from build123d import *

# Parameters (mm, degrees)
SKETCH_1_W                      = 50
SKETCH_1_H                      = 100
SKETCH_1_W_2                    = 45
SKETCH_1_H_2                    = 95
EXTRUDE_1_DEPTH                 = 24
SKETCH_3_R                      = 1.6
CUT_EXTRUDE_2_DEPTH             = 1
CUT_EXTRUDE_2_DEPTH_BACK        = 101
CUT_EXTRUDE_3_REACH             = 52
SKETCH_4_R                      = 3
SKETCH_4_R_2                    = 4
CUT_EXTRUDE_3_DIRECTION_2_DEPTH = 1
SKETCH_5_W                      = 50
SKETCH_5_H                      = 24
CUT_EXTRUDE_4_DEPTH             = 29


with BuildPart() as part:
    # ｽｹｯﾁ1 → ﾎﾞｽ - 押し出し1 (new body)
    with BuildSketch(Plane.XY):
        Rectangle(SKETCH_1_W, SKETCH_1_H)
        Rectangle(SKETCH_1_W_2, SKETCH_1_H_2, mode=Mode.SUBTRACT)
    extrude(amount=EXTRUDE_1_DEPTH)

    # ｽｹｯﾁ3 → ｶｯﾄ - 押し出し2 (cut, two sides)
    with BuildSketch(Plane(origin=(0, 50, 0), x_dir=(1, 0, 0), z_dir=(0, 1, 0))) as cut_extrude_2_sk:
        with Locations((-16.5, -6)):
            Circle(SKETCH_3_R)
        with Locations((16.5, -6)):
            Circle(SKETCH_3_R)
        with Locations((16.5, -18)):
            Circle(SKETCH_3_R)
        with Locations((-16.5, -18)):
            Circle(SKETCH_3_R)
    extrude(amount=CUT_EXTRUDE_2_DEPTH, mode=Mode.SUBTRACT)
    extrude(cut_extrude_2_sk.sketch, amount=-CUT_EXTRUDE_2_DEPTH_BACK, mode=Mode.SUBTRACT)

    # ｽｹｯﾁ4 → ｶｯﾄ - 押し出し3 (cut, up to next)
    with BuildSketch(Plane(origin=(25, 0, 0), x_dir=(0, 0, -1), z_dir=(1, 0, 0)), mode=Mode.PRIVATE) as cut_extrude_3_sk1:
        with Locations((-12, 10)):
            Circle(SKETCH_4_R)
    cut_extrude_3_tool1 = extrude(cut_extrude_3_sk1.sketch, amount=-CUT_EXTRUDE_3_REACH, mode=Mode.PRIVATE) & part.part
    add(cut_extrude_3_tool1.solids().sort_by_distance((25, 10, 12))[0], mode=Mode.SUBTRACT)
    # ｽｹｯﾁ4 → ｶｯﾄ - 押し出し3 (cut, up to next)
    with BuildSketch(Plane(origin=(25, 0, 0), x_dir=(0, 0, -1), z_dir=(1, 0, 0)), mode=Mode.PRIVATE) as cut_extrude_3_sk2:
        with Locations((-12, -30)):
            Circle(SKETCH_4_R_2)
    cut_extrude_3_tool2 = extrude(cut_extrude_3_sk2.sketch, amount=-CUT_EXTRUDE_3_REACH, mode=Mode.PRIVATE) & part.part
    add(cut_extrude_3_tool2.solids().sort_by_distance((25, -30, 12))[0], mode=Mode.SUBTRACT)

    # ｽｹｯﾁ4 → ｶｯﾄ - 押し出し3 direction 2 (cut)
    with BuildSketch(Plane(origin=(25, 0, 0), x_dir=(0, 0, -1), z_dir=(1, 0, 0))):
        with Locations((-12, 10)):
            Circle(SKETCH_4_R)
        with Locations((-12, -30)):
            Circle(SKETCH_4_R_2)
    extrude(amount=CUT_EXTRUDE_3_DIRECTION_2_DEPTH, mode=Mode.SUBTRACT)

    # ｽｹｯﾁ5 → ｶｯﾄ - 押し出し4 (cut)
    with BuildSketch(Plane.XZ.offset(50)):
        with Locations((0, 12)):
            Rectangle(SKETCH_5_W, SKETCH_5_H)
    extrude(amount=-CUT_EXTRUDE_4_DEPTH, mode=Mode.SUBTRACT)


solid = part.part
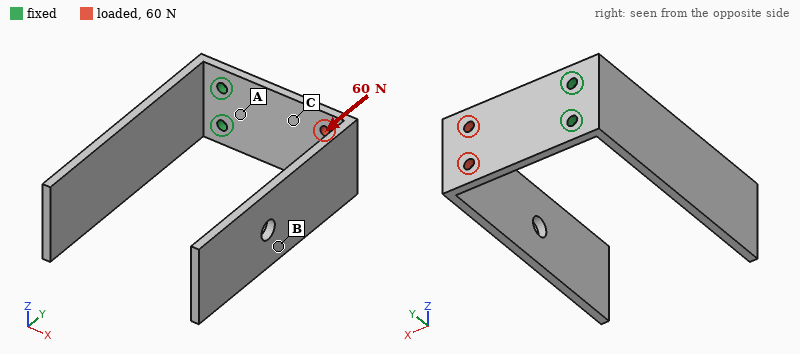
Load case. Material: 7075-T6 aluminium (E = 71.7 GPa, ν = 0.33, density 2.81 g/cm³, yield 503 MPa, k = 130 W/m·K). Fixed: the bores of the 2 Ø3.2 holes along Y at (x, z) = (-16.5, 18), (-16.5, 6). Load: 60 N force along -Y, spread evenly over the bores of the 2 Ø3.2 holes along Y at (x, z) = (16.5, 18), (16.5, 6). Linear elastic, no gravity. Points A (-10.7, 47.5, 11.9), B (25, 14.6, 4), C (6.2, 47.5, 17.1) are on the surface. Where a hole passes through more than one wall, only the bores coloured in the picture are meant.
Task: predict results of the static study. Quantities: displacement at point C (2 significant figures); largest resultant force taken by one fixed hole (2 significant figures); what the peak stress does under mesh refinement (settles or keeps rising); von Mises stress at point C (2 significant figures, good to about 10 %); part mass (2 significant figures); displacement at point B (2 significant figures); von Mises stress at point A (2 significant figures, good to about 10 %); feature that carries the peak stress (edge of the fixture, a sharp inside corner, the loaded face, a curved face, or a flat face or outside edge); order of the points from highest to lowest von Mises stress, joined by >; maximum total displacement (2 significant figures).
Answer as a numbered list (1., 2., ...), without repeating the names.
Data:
1. 0.16 mm
2. 30 N
3. keeps rising
4. 24 MPa
5. 31 g
6. 0.62 mm
7. 59 MPa
8. edge of the fixture
9. A > C > B
10. 1.0 mm
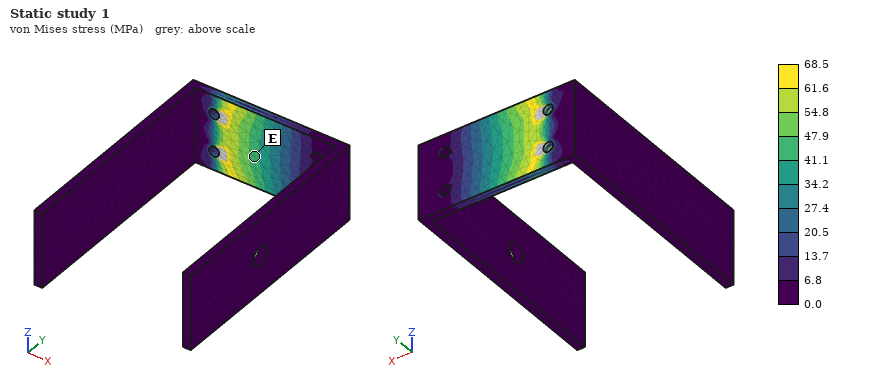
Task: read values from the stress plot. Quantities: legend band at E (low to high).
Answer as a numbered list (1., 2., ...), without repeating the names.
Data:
1. 41.1 to 47.9 MPa
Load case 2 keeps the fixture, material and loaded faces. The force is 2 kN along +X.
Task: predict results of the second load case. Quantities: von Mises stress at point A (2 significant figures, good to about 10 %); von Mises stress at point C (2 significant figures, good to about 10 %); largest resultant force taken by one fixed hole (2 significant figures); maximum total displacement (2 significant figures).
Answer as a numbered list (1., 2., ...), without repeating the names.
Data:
1. 28 MPa
2. 35 MPa
3. 1.0 kN
4. 21 µm
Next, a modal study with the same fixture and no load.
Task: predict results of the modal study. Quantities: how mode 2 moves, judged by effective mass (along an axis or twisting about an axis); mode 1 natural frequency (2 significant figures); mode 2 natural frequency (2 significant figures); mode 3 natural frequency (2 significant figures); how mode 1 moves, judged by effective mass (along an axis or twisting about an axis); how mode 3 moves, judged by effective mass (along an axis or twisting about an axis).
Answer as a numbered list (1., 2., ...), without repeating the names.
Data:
1. along Z
2. 220 Hz
3. 360 Hz
4. 370 Hz
5. along X
6. along X
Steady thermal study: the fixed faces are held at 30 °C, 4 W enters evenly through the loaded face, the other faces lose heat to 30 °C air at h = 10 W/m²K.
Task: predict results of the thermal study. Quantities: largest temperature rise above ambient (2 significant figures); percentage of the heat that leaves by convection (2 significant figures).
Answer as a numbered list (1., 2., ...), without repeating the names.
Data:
1. 15 K
2. 17 %
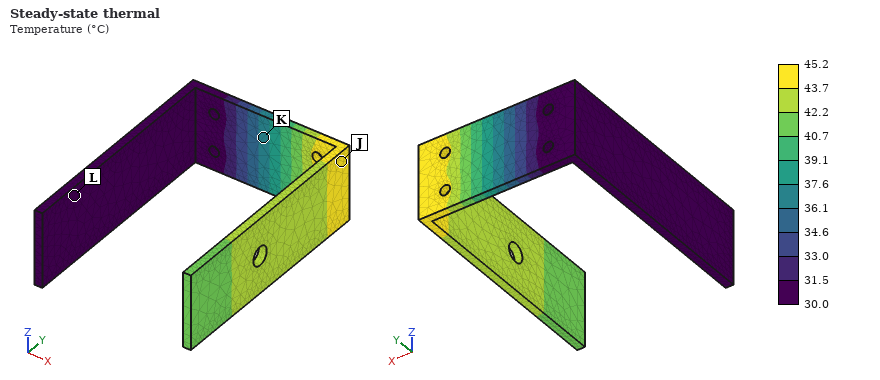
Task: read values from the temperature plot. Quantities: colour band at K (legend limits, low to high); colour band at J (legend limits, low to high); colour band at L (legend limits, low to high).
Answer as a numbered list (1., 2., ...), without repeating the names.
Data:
1. 36.1 to 37.6 °C
2. 43.7 to 45.2 °C
3. 30.0 to 31.5 °C
